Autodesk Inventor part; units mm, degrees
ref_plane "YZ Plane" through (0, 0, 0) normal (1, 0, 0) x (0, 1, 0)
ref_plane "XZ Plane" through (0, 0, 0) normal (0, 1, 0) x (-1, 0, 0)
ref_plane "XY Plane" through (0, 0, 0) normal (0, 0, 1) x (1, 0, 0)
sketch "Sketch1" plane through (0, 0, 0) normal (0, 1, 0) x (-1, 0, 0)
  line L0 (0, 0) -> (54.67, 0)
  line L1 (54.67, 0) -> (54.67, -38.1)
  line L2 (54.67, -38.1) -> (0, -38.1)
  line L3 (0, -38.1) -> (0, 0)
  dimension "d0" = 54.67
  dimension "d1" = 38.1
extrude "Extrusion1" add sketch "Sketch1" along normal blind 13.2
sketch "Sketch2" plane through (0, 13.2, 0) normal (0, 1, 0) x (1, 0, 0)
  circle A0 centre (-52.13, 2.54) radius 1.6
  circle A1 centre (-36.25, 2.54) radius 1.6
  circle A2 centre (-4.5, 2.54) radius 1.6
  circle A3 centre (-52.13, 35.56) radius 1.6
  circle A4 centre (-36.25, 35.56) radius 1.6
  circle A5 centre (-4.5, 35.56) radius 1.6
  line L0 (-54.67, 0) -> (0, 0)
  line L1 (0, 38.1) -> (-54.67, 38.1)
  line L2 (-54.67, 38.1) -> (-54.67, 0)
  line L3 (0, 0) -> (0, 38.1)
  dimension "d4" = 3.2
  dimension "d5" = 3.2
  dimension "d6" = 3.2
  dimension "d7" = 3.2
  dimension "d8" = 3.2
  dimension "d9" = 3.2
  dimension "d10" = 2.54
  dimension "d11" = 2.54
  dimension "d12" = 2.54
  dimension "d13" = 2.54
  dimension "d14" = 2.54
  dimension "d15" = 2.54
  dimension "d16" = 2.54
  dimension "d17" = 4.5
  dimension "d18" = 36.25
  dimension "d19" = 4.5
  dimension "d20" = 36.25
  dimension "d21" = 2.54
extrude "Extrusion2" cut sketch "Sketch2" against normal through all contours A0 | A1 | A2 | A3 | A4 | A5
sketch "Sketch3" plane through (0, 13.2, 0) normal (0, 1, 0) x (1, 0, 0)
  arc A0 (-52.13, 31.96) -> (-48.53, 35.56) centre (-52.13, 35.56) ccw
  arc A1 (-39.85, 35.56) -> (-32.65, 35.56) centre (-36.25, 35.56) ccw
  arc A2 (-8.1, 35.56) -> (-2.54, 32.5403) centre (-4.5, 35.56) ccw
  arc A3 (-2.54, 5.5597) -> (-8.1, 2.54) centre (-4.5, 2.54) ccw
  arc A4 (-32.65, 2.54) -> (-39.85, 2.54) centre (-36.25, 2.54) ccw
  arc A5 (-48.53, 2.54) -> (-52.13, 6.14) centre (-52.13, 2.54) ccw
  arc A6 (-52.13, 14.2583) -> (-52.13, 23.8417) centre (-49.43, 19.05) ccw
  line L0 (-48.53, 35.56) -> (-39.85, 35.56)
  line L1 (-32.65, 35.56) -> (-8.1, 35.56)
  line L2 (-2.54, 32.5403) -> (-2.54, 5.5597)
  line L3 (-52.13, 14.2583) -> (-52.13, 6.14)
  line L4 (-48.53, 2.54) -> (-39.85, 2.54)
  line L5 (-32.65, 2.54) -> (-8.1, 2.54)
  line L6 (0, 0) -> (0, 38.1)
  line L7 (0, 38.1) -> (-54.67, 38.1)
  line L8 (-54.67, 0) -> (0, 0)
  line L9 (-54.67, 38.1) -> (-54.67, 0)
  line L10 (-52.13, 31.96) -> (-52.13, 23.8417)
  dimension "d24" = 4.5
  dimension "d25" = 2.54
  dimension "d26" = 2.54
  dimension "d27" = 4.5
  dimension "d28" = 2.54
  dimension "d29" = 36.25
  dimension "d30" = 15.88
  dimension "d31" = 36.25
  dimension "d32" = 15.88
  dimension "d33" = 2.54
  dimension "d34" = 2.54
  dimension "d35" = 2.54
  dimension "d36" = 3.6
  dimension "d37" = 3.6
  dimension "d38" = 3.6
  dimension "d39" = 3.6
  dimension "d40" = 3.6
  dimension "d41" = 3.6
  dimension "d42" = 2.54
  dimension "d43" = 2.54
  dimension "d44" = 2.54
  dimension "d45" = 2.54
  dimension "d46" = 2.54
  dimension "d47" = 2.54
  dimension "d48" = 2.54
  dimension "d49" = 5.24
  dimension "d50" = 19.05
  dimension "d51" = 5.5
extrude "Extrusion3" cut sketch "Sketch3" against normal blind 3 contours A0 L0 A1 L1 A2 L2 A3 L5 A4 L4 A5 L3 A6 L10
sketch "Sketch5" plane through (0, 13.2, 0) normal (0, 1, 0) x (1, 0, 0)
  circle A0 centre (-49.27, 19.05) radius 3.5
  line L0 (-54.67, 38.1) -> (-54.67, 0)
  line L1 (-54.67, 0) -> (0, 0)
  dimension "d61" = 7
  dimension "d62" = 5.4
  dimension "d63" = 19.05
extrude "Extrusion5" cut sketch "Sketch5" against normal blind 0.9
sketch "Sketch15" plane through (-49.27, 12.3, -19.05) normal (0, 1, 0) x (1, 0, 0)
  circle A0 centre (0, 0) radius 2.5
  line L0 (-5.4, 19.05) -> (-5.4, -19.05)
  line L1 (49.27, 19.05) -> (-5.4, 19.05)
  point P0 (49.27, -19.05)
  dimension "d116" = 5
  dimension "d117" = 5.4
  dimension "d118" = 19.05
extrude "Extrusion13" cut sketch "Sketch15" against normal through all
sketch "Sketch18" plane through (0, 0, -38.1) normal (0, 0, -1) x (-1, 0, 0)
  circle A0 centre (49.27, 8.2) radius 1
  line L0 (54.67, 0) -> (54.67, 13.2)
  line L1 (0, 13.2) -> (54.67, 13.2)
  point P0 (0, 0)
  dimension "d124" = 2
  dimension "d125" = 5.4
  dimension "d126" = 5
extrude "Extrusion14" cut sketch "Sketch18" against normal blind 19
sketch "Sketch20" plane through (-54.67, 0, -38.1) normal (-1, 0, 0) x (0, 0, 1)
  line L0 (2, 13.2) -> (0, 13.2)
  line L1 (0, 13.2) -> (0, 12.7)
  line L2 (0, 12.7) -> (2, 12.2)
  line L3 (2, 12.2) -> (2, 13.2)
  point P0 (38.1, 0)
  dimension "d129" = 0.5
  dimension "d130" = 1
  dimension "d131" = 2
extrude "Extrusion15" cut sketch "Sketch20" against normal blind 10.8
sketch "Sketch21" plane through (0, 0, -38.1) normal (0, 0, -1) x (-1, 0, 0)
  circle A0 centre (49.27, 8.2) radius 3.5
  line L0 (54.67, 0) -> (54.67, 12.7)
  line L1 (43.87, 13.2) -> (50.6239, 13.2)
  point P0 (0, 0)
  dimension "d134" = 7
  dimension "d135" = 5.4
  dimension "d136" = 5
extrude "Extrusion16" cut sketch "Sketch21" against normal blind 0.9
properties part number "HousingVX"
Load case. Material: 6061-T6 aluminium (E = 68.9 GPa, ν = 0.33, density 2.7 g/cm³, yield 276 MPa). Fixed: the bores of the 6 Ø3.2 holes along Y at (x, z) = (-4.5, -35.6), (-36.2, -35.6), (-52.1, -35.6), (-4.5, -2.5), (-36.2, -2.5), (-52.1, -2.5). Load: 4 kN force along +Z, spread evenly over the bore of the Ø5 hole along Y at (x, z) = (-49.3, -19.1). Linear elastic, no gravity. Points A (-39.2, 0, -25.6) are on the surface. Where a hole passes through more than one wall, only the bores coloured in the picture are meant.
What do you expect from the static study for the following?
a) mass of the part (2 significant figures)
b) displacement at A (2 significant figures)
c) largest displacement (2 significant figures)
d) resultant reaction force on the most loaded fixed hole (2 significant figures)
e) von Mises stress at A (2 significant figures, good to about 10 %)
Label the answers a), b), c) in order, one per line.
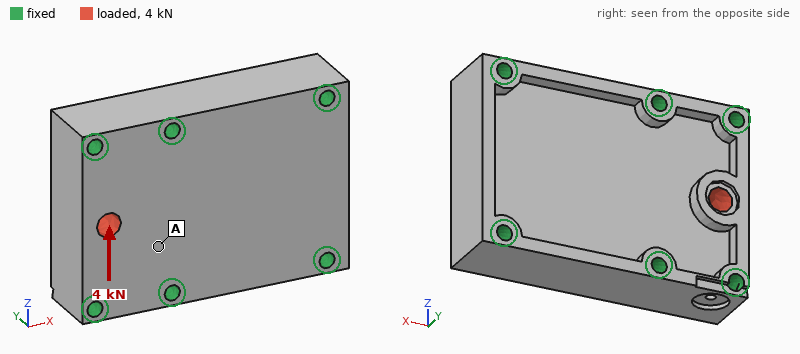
a) 60 g
b) 0.87 µm
c) 4.5 µm
d) 1.4 kN
e) 4.8 MPa
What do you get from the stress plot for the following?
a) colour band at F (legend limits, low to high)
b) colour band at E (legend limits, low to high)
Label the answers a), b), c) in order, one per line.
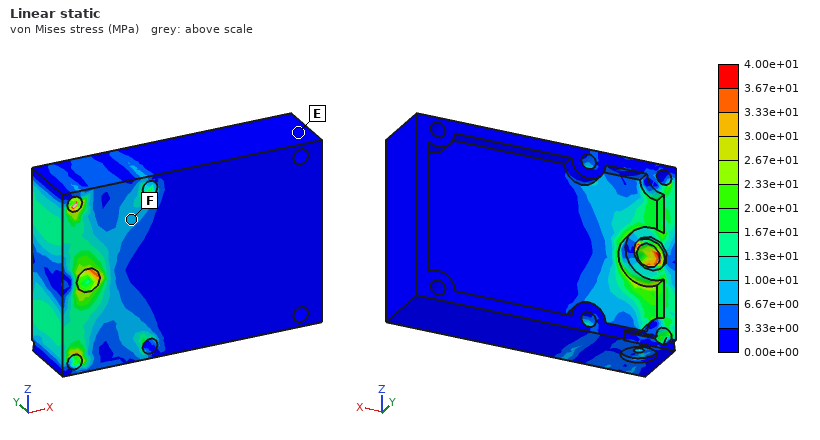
a) 6.67e+00 to 1.00e+01 MPa
b) 0.00e+00 to 3.33e+00 MPa
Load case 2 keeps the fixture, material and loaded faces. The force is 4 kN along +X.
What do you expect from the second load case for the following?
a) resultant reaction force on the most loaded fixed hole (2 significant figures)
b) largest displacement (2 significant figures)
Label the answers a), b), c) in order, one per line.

a) 1.2 kN
b) 10 µm
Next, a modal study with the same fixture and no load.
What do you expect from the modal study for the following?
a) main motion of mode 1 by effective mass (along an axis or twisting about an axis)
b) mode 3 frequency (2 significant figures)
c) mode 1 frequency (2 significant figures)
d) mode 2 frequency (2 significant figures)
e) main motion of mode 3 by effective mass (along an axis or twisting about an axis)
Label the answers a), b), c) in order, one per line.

a) along Y
b) 38 kHz
c) 25 kHz
d) 34 kHz
e) along Z
